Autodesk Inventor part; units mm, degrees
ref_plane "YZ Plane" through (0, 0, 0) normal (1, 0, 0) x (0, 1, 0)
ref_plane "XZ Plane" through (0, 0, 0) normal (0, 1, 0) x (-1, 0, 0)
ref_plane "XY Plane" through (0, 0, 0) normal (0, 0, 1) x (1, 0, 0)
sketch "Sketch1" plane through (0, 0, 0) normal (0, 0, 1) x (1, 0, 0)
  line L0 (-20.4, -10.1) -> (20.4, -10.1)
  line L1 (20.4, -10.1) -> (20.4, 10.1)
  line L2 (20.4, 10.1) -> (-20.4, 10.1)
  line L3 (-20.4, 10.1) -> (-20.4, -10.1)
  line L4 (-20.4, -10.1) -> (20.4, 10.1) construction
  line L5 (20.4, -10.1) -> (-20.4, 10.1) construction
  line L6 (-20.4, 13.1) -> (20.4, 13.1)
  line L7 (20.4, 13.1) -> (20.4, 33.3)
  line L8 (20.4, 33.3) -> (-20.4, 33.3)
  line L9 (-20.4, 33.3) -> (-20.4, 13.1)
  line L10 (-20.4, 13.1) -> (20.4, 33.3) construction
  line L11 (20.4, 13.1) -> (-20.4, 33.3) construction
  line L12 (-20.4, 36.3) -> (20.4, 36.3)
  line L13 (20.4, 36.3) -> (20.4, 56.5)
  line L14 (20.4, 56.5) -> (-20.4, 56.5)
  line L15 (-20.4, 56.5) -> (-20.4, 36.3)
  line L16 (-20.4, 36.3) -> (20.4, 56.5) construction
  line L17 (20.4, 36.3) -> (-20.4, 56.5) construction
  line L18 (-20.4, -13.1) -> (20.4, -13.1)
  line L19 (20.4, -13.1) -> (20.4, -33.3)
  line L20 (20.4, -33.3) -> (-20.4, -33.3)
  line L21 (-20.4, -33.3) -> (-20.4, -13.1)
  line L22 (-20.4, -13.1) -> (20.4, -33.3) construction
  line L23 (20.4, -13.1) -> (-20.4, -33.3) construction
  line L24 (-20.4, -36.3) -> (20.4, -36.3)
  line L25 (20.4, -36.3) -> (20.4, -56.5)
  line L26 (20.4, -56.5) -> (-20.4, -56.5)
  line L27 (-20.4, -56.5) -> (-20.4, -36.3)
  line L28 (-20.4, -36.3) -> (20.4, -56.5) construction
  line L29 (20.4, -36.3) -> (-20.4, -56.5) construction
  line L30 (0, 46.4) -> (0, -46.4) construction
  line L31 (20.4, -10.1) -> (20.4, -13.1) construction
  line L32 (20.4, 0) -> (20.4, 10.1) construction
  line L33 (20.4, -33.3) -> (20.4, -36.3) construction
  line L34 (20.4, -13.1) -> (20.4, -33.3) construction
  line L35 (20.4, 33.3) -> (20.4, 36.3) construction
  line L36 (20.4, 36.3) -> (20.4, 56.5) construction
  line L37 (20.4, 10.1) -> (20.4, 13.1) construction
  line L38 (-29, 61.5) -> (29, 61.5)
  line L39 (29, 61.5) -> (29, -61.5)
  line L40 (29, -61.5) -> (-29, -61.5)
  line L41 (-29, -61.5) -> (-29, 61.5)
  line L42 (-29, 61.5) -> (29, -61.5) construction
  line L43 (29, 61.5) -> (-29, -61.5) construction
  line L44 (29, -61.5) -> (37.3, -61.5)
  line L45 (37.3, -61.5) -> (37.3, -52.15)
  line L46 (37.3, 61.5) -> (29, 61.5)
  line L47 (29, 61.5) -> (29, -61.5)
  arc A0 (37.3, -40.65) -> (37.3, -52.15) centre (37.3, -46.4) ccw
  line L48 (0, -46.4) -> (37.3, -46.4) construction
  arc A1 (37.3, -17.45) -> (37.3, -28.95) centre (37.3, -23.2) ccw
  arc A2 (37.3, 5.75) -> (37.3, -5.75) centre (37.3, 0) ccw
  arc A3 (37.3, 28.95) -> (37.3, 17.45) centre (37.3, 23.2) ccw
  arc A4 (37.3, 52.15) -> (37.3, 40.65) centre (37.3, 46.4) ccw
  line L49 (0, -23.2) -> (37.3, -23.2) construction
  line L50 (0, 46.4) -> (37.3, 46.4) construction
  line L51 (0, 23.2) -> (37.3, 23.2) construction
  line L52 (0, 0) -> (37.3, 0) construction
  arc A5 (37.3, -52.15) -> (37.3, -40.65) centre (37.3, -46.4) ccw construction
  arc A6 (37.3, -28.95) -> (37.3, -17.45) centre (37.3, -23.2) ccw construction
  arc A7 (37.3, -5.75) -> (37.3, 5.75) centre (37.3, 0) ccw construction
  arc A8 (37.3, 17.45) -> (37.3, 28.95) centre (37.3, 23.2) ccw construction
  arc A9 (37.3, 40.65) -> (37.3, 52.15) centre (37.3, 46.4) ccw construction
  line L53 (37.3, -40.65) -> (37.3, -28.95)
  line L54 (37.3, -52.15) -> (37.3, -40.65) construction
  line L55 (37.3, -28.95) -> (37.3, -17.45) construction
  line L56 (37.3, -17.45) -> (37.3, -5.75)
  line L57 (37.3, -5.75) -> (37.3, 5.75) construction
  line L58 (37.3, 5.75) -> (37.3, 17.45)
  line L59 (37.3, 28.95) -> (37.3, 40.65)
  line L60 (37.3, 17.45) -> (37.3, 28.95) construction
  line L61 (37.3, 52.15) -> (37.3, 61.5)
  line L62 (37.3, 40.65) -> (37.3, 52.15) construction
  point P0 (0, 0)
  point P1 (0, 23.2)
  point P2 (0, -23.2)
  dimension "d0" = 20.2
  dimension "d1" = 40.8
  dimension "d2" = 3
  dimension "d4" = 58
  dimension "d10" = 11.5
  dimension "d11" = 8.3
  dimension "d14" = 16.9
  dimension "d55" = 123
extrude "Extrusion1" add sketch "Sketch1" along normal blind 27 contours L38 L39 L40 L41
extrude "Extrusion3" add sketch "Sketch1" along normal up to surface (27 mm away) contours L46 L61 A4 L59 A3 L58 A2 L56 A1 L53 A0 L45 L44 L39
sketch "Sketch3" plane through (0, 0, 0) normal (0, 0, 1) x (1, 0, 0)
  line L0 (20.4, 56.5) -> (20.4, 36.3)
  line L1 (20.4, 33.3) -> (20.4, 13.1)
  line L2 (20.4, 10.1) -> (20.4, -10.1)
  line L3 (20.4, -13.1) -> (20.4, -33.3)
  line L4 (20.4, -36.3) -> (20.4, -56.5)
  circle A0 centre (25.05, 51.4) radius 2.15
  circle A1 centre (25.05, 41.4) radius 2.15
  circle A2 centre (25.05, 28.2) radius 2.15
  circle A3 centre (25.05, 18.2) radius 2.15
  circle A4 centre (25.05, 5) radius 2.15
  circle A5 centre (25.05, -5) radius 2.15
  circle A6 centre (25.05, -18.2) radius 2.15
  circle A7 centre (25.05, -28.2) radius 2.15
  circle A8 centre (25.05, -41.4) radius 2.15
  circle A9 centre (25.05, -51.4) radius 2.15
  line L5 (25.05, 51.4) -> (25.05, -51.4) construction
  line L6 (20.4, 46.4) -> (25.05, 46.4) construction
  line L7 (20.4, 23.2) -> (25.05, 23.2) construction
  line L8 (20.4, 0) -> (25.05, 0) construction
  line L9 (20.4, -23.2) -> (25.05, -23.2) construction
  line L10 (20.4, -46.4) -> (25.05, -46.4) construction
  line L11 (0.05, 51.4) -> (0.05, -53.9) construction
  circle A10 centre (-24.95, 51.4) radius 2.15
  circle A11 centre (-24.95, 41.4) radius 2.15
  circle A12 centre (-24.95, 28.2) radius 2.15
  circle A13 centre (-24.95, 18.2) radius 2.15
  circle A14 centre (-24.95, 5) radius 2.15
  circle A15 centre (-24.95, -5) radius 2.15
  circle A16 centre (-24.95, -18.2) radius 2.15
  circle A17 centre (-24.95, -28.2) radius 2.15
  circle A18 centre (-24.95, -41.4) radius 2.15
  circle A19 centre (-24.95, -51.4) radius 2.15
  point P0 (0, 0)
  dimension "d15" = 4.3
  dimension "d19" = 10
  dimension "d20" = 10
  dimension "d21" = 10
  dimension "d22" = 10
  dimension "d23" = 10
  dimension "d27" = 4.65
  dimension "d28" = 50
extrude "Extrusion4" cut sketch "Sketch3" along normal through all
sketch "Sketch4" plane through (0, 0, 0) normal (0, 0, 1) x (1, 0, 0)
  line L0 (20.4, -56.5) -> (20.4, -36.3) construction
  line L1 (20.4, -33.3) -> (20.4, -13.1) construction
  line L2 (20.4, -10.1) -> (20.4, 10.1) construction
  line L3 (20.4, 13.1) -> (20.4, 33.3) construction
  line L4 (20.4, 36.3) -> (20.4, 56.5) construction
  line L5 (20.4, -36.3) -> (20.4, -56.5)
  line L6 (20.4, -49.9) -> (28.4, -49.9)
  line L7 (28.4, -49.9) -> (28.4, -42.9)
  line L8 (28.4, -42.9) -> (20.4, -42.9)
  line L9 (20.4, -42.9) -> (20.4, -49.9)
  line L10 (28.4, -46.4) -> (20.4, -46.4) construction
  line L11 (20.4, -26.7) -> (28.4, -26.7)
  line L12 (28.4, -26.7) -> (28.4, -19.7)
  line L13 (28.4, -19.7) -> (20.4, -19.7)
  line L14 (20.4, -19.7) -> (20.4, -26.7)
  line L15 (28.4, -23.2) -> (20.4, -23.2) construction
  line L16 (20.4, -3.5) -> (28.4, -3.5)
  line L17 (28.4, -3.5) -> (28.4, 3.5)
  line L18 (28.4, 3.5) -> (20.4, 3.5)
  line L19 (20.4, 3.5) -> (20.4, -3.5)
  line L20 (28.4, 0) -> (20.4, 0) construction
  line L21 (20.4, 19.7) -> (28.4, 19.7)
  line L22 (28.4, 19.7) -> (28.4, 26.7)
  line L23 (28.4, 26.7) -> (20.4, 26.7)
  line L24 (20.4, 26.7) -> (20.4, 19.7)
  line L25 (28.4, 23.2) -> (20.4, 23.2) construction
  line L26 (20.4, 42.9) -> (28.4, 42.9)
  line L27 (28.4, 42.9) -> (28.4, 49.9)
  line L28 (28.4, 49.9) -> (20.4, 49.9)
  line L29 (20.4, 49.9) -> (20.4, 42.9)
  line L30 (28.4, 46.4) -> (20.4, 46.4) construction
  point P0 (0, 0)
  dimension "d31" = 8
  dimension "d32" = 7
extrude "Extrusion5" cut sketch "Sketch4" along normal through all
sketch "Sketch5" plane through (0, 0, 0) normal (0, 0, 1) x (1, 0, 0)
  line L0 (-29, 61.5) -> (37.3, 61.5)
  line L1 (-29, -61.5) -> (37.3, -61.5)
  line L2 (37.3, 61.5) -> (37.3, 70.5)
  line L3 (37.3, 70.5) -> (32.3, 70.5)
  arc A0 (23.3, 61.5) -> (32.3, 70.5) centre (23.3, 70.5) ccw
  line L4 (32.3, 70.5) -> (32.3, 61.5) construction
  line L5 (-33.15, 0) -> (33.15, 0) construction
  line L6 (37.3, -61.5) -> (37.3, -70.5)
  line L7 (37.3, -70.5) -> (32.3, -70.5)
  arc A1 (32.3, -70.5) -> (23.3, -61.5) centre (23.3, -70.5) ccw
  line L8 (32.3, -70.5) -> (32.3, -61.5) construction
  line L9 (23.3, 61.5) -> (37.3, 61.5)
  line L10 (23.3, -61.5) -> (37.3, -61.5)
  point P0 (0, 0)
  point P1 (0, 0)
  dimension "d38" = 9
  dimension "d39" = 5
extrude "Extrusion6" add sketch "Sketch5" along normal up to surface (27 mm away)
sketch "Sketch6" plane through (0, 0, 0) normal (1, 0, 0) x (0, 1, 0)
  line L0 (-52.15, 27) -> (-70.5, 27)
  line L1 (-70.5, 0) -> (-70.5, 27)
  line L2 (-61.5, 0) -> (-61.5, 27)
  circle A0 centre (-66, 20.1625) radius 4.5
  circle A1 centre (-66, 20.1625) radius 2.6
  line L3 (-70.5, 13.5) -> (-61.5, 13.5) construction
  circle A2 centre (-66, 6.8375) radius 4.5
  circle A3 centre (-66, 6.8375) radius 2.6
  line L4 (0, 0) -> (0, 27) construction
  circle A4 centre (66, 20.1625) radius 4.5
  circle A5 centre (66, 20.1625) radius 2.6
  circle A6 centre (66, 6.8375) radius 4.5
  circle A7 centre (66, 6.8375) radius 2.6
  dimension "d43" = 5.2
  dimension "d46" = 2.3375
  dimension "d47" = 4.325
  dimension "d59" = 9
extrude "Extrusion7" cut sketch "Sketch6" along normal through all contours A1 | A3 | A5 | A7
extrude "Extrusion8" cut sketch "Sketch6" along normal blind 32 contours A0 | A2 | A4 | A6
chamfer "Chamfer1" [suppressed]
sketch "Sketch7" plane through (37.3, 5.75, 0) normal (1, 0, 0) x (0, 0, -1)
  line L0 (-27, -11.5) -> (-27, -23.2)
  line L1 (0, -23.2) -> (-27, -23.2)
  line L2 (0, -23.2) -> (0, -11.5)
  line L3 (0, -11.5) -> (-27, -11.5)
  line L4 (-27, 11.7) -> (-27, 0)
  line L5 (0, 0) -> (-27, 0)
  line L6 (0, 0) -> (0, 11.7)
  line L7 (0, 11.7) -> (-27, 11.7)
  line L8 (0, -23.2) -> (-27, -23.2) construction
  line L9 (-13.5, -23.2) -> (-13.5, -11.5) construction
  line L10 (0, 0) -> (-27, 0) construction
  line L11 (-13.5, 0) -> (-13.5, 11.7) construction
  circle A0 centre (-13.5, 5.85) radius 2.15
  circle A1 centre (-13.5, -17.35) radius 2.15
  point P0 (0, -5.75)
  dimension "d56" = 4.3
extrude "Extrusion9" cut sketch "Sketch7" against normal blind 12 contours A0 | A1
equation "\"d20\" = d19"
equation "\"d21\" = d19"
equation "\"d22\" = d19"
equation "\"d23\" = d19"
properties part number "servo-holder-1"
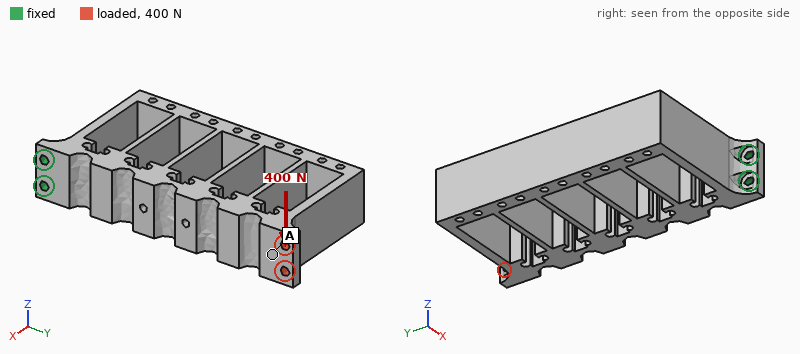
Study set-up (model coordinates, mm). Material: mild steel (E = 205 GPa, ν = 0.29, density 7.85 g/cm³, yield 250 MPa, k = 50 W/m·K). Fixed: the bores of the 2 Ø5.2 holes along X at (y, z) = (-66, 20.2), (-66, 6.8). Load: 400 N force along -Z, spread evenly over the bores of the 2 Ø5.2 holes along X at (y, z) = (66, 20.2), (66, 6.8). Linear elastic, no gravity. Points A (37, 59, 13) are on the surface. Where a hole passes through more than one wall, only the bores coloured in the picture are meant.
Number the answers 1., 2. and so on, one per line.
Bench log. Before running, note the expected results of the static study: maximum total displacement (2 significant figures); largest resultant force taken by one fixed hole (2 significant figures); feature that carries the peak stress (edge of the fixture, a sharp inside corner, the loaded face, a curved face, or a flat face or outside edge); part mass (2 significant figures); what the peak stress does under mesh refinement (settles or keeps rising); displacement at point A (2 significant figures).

1. 0.18 mm
2. 3.1 kN
3. edge of the fixture
4. 700 g
5. keeps rising
6. 0.16 mm
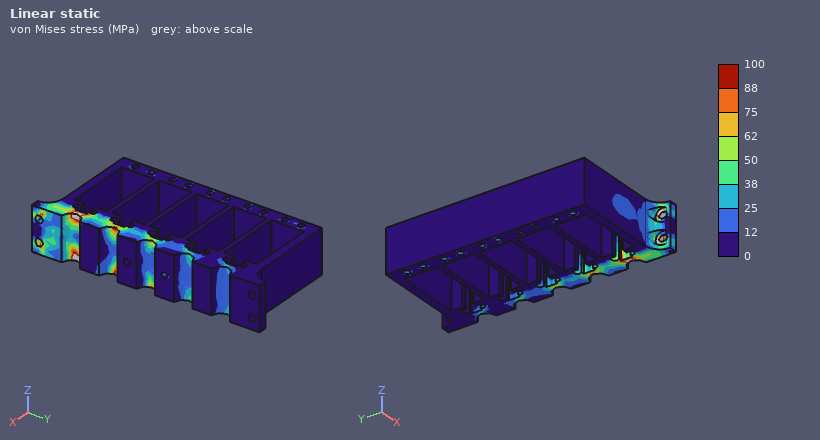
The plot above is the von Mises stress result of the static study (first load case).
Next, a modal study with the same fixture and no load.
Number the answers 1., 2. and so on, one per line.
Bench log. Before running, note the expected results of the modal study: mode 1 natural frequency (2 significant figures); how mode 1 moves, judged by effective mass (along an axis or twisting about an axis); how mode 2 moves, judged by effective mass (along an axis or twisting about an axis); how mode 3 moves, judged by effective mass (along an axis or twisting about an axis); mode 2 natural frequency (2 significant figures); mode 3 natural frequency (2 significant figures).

1. 220 Hz
2. along X
3. along Z
4. twisting about Y
5. 480 Hz
6. 1000 Hz
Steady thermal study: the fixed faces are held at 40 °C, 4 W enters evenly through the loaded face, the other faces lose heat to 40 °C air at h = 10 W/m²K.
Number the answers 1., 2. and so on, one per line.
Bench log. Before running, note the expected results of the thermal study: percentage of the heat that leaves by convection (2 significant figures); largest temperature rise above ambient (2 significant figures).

1. 77 %
2. 24 K
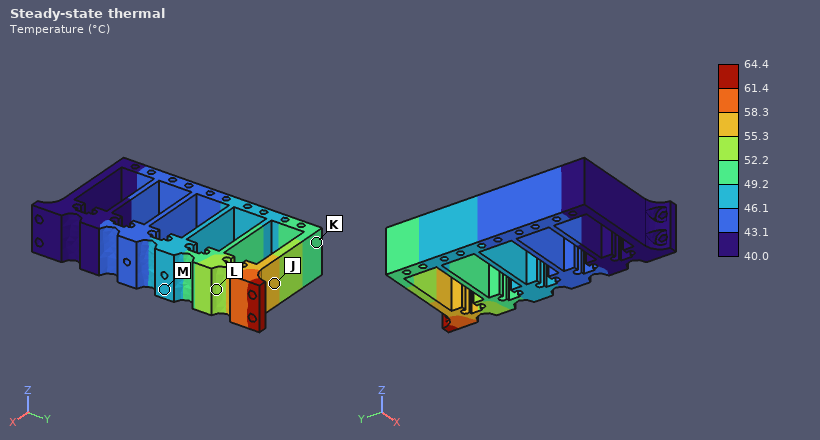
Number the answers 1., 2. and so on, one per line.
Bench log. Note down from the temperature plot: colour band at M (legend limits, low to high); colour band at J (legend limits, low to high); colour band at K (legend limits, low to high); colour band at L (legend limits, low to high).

1. 46.1 to 49.2 °C
2. 55.3 to 58.3 °C
3. 49.2 to 52.2 °C
4. 52.2 to 55.3 °C
